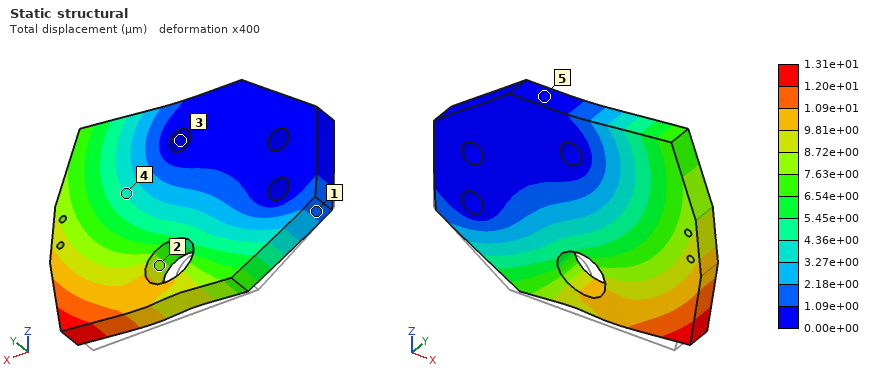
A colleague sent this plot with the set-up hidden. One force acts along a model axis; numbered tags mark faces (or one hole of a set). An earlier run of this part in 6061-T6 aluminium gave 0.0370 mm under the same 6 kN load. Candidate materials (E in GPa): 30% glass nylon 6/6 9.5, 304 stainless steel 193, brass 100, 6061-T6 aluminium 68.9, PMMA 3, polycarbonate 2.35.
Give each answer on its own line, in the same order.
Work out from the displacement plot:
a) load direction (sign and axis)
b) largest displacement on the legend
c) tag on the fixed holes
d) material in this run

+X
1.31e+01 µm
3
304 stainless steel
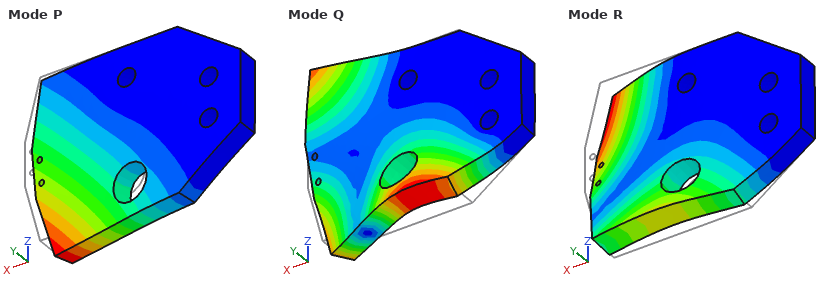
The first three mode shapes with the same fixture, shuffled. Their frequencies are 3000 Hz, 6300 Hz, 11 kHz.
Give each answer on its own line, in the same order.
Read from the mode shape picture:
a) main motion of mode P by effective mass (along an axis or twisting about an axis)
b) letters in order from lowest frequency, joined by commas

along Y
P, R, Q
